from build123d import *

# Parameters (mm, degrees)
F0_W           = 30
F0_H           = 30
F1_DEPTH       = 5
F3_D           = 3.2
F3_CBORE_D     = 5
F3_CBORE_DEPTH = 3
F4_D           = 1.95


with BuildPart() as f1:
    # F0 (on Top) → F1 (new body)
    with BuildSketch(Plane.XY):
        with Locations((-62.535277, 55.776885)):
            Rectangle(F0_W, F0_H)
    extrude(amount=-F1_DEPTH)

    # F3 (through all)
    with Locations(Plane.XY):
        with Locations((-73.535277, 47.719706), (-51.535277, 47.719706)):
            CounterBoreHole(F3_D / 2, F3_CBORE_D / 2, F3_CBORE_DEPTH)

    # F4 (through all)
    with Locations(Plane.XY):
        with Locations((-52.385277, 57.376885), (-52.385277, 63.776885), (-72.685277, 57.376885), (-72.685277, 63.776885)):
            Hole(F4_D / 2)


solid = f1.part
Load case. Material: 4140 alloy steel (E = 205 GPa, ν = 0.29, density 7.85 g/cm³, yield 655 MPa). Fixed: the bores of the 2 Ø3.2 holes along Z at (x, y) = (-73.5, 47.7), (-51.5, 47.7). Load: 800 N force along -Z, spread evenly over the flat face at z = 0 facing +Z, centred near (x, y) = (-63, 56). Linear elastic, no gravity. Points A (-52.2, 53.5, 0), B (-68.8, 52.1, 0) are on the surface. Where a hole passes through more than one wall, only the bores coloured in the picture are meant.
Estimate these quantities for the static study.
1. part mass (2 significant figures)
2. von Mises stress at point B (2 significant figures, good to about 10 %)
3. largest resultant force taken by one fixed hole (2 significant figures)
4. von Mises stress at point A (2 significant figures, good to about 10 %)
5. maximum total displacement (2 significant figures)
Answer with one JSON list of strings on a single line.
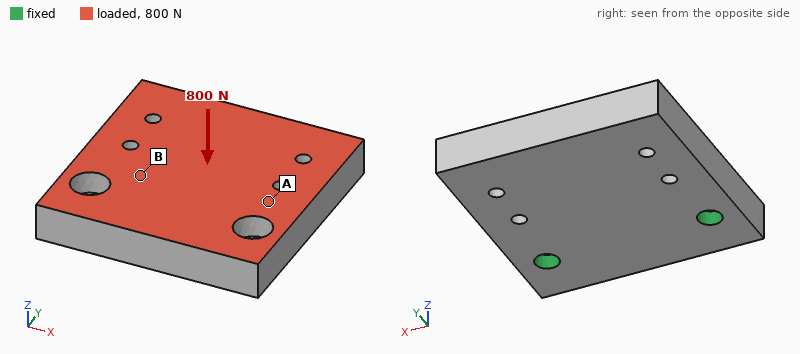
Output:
["34 g", "48 MPa", "440 N", "25 MPa", "46 µm"]
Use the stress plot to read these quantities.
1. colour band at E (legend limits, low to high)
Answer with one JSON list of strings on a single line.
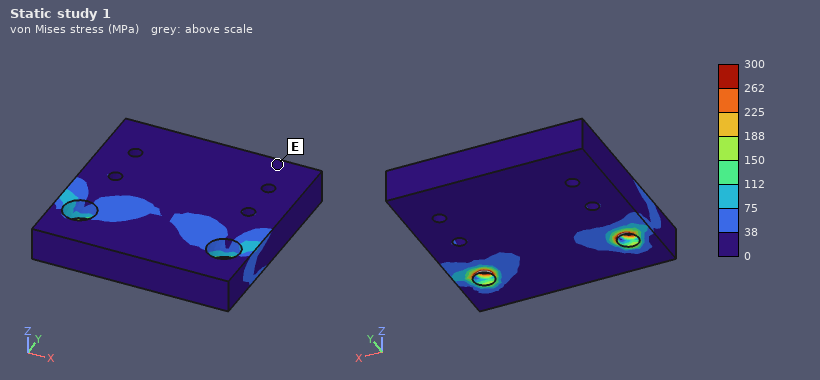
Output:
["0 to 38 MPa"]
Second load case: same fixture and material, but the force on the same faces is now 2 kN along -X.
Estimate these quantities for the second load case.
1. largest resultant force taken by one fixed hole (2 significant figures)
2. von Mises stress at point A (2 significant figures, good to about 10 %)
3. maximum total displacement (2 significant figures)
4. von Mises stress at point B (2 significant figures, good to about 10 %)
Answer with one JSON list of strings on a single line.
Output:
["1.3 kN", "24 MPa", "7.0 µm", "21 MPa"]
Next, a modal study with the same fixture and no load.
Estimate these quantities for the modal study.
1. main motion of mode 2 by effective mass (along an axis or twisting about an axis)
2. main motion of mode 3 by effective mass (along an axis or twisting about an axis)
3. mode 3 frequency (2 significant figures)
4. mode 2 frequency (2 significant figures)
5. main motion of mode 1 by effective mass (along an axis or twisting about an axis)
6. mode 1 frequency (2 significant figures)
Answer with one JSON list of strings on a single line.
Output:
["twisting about Y", "along X", "21 kHz", "12 kHz", "along Z", "4400 Hz"]
